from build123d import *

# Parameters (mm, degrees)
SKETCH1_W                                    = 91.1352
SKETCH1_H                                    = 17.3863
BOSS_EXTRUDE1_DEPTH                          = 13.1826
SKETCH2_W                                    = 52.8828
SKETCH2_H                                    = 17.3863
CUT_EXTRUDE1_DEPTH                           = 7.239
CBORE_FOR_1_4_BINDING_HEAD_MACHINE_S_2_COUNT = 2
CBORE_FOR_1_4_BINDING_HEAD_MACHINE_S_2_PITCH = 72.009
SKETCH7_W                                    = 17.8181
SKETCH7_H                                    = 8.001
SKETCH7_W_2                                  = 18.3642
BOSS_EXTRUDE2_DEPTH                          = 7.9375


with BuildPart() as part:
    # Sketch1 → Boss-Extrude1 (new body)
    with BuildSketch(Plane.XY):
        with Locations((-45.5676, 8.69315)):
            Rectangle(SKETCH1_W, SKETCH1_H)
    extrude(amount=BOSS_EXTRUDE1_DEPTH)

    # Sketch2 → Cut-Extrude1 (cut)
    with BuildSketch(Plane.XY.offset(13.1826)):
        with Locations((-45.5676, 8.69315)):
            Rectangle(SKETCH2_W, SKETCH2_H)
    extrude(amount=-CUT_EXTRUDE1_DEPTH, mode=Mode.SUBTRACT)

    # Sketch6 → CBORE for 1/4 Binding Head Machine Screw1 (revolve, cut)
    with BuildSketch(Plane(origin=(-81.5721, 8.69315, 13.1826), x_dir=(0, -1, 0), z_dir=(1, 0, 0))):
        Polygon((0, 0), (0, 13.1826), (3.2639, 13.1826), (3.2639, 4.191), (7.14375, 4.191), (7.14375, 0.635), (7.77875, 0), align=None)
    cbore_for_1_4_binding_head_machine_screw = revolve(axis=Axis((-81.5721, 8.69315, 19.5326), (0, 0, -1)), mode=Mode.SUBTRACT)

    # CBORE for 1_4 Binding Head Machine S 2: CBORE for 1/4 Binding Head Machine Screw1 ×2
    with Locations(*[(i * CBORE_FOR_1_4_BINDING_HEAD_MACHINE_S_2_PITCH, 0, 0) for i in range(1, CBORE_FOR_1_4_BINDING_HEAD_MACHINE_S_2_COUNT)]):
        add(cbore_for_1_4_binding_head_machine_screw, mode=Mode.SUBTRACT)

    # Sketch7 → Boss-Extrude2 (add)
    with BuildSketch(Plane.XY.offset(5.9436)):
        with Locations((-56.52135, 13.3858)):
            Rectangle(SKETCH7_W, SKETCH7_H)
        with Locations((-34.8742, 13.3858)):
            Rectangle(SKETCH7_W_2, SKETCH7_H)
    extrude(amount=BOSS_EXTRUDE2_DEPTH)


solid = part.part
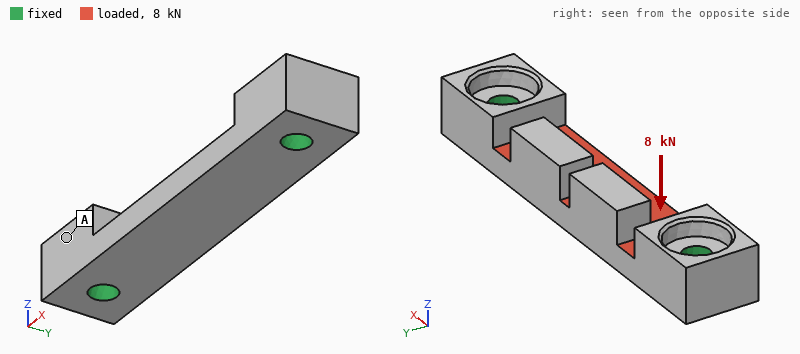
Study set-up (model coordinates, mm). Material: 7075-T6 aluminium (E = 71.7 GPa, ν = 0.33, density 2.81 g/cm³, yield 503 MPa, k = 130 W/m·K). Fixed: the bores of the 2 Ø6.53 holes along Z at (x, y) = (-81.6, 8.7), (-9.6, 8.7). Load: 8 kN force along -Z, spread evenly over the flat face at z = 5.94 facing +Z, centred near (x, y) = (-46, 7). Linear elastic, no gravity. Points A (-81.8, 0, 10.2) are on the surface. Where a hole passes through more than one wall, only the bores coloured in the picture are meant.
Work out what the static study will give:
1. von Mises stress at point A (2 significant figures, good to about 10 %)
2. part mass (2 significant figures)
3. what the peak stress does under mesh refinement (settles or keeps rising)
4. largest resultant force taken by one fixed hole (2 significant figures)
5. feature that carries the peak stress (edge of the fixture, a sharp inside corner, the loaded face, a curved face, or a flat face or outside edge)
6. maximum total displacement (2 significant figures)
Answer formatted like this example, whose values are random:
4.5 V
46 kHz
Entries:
45 MPa
41 g
keeps rising
4.0 kN
edge of the fixture
0.27 mm
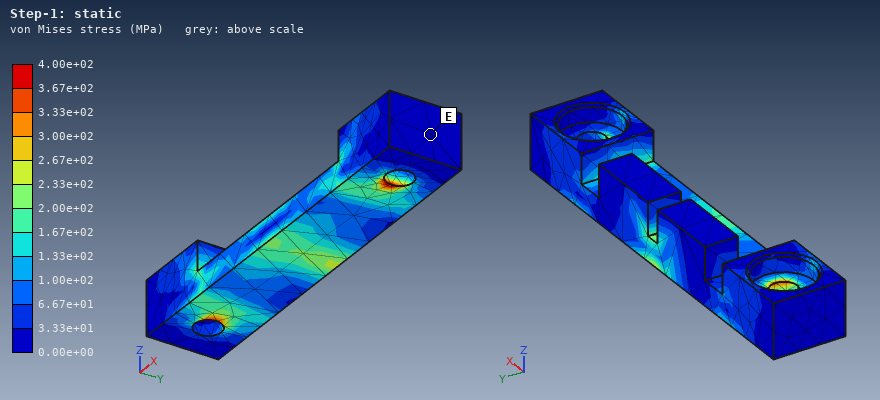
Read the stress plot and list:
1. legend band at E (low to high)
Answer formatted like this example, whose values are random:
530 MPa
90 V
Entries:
0.00e+00 to 3.33e+01 MPa
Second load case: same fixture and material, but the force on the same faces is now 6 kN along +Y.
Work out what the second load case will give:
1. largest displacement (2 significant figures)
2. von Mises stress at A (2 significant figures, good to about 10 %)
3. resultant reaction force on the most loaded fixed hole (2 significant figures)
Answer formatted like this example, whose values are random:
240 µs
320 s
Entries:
0.10 mm
22 MPa
3.0 kN
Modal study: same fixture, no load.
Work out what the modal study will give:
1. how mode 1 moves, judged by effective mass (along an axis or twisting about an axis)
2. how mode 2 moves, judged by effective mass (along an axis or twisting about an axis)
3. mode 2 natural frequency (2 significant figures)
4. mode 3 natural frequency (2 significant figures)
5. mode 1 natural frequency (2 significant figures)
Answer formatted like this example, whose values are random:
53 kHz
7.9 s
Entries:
along Z
along Y
9700 Hz
14 kHz
6900 Hz
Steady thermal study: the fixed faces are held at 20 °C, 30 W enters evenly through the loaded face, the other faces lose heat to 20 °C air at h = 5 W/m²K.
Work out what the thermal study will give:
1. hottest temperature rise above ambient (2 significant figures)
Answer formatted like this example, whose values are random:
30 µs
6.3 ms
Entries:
20 K
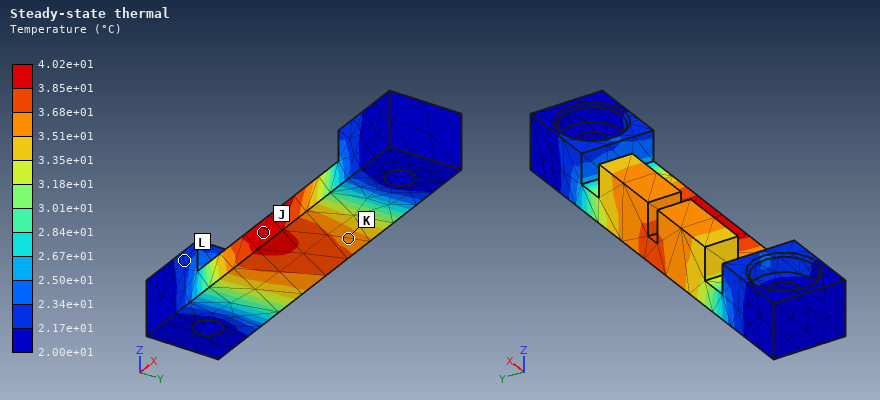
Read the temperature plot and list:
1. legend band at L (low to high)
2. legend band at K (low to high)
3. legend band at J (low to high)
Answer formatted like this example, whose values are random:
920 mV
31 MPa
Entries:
2.17e+01 to 2.34e+01 °C
3.51e+01 to 3.68e+01 °C
3.85e+01 to 4.02e+01 °C
